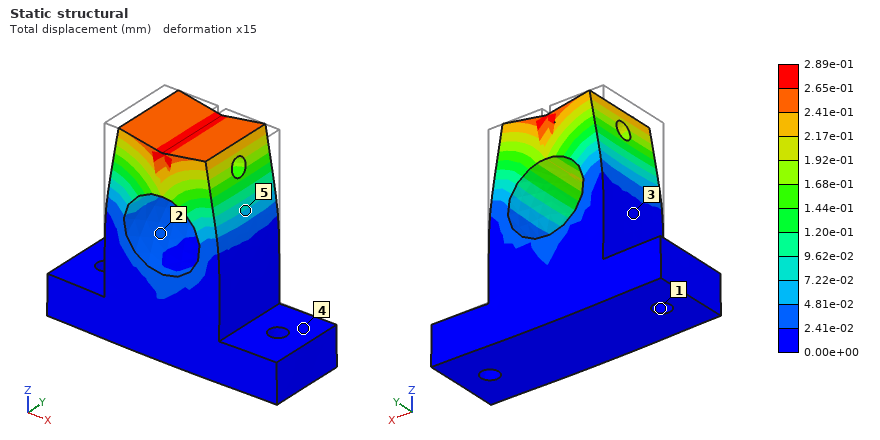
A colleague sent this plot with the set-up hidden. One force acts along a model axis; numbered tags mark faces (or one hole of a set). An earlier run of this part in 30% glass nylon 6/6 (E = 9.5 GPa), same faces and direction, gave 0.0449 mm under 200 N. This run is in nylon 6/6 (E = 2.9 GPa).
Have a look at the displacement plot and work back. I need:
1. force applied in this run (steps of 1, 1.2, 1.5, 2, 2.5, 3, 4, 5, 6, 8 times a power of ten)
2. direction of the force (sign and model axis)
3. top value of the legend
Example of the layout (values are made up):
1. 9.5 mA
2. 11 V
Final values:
1. 400 N
2. -Z
3. 2.89e-01 mm
